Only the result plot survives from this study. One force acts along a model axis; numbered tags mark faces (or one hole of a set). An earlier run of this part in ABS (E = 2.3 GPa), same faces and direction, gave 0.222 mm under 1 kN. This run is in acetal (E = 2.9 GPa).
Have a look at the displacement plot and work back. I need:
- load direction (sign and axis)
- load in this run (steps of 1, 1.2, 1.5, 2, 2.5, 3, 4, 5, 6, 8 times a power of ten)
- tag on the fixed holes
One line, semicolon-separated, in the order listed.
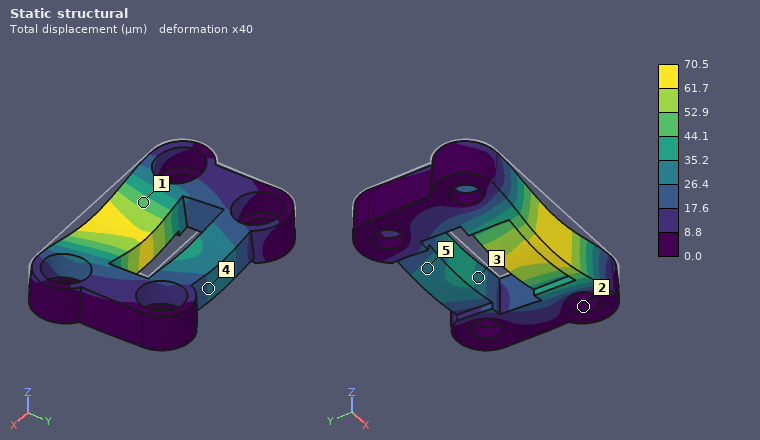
-Z; 400 N; 2
